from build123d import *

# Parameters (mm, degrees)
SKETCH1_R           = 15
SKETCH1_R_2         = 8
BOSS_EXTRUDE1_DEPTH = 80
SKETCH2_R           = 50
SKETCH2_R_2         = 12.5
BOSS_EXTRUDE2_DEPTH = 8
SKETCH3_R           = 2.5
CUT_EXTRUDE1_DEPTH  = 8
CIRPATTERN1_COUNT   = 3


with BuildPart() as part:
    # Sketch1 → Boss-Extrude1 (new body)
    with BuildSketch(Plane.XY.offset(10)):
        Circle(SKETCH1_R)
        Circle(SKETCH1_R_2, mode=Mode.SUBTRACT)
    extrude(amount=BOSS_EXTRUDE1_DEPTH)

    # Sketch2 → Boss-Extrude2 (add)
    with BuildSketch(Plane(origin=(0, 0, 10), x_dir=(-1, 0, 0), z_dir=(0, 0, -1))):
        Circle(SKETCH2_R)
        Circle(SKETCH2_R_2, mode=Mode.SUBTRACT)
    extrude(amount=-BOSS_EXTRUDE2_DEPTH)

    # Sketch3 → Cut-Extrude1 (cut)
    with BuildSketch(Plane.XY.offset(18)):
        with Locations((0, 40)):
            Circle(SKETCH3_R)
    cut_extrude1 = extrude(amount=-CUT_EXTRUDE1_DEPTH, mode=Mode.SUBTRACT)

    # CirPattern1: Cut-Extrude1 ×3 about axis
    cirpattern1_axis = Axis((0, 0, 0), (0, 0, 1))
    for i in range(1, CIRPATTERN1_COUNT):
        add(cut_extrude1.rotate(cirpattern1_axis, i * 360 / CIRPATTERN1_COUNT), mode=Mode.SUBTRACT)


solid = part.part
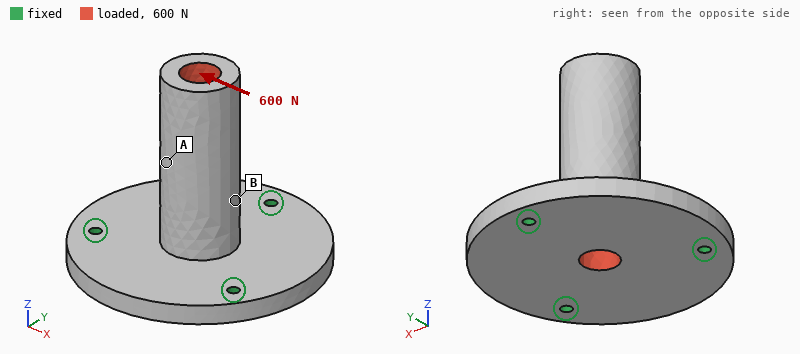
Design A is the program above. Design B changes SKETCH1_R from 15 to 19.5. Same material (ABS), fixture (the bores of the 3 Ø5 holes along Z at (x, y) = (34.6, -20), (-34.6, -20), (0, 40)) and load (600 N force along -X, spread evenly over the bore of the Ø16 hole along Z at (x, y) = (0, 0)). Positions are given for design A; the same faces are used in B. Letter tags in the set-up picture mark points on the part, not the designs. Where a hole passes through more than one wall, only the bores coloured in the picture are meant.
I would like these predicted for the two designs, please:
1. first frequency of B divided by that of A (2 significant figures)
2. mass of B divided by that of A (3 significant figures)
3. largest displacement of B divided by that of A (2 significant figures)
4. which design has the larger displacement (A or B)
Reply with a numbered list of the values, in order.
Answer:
1. 0.97
2. 1.36
3. 0.53
4. A
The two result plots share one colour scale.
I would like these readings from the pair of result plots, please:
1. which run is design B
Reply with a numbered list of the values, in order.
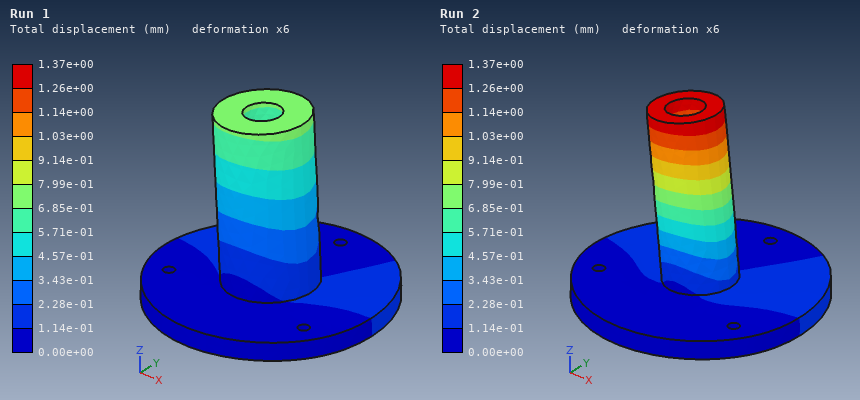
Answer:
1. Run 1
